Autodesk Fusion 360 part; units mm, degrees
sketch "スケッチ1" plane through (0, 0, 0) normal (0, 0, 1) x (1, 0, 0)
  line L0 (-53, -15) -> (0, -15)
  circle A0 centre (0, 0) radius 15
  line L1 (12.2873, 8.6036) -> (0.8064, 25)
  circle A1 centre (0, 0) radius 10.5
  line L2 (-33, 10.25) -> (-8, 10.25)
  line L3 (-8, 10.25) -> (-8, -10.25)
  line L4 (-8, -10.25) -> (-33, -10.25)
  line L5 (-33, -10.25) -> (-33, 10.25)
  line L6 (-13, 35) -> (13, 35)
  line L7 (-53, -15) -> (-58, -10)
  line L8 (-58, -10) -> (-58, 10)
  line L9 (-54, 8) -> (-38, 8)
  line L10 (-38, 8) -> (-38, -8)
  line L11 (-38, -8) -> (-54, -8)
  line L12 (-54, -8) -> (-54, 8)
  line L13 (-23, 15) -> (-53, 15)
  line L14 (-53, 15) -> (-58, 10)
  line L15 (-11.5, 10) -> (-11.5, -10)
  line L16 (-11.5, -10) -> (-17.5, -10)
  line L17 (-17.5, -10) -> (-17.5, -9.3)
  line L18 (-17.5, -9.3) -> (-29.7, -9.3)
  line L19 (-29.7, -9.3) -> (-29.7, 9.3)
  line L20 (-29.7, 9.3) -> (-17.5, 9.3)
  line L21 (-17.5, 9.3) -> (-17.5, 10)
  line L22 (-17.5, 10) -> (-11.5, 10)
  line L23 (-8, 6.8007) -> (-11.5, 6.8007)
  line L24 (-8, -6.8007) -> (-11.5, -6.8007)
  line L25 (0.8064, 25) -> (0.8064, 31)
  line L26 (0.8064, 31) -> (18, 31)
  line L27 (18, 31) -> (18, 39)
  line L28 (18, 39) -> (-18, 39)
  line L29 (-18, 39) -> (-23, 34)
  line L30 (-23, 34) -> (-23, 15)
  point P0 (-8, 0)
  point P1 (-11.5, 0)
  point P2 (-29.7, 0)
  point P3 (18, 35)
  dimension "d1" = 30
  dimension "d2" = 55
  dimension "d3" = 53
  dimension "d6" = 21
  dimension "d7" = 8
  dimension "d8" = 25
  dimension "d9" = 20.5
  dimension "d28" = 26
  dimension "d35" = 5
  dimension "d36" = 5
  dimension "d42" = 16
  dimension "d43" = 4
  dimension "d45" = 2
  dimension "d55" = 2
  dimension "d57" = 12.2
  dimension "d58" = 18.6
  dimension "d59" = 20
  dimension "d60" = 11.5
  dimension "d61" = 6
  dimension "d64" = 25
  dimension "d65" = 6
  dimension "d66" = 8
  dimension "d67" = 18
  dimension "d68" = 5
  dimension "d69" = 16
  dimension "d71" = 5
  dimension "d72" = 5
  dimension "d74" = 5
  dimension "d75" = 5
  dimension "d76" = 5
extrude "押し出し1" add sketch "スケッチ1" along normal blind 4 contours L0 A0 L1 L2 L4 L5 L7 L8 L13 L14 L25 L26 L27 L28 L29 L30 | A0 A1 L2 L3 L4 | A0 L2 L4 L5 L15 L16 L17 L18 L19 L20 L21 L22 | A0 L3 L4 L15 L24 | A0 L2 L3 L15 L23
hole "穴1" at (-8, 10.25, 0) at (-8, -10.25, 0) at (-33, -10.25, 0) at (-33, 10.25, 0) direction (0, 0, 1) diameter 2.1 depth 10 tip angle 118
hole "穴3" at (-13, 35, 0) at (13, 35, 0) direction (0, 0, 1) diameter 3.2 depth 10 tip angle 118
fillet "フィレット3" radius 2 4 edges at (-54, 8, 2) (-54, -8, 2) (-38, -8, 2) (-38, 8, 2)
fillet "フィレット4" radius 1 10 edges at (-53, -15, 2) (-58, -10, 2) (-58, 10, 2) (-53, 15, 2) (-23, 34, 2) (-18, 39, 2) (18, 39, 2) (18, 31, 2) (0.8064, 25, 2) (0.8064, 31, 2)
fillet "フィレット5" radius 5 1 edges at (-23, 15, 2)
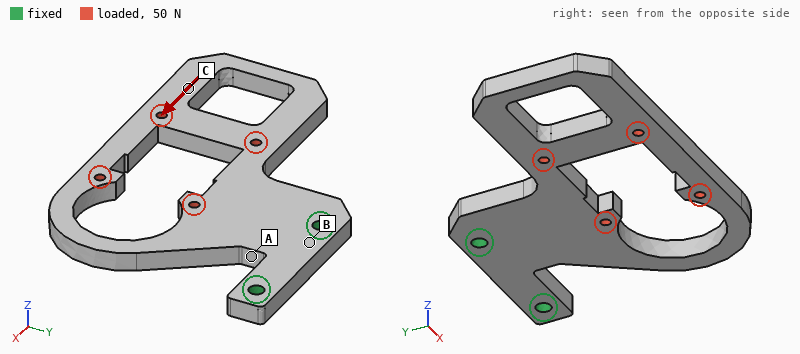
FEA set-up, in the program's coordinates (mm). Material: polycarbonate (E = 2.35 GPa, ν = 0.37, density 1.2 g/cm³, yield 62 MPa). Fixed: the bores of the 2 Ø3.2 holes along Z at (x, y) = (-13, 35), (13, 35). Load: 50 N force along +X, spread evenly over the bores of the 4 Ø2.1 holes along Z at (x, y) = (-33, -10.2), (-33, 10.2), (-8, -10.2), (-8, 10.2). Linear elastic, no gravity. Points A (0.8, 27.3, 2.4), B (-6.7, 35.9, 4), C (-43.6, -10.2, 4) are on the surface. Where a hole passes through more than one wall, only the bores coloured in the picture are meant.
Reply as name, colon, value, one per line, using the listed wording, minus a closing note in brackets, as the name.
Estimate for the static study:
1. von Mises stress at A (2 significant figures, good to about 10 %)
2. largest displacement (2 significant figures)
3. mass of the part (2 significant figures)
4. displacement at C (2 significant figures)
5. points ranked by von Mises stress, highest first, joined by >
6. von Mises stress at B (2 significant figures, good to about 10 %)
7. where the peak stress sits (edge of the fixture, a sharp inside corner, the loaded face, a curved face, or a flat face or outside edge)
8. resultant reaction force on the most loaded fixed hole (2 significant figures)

von Mises stress at A: 5.2 MPa
largest displacement: 1.0 mm
mass of the part: 8.7 g
displacement at C: 0.80 mm
points ranked by von Mises stress, highest first, joined by >: A > B > C
von Mises stress at B: 3.1 MPa
where the peak stress sits: a curved face
resultant reaction force on the most loaded fixed hole: 65 N
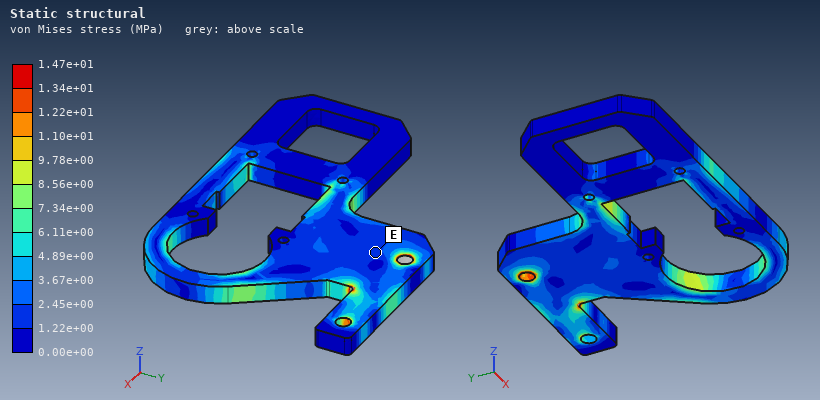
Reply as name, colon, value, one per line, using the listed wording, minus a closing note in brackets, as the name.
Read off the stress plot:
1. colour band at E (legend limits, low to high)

colour band at E: 1.22e+00 to 2.45e+00 MPa
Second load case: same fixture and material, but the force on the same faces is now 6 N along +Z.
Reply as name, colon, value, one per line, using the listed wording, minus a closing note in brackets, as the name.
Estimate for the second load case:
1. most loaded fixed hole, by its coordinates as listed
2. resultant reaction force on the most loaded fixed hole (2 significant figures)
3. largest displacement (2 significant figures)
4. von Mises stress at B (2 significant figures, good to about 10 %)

most loaded fixed hole, by its coordinates as listed: (-13, 35)
resultant reaction force on the most loaded fixed hole: 8.1 N
largest displacement: 0.93 mm
von Mises stress at B: 0.93 MPa
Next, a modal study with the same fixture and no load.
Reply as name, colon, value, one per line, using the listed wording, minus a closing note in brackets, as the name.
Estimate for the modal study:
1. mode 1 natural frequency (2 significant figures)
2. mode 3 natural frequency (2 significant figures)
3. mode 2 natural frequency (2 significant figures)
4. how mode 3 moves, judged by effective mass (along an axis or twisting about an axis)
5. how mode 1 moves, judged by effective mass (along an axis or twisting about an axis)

mode 1 natural frequency: 200 Hz
mode 3 natural frequency: 520 Hz
mode 2 natural frequency: 360 Hz
how mode 3 moves, judged by effective mass: along X
how mode 1 moves, judged by effective mass: along Z
